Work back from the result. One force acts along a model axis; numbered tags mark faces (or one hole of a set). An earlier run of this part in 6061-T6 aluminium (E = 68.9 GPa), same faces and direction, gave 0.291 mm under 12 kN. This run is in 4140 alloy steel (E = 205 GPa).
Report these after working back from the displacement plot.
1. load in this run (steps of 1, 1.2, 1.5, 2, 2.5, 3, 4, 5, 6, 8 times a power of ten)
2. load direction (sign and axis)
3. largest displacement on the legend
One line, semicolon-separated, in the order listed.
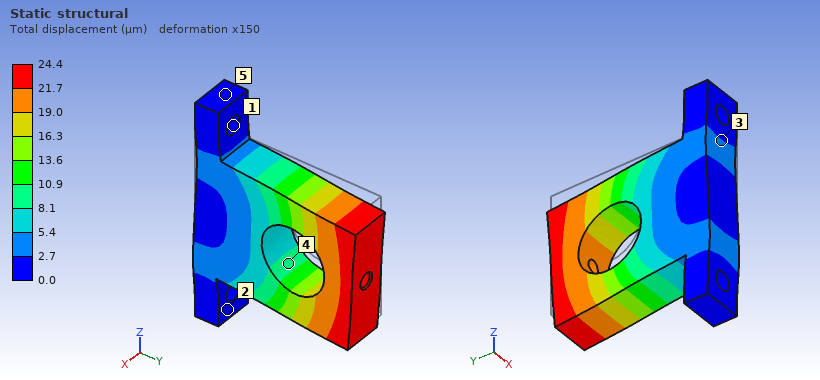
3 kN; -Z; 24.4 µm
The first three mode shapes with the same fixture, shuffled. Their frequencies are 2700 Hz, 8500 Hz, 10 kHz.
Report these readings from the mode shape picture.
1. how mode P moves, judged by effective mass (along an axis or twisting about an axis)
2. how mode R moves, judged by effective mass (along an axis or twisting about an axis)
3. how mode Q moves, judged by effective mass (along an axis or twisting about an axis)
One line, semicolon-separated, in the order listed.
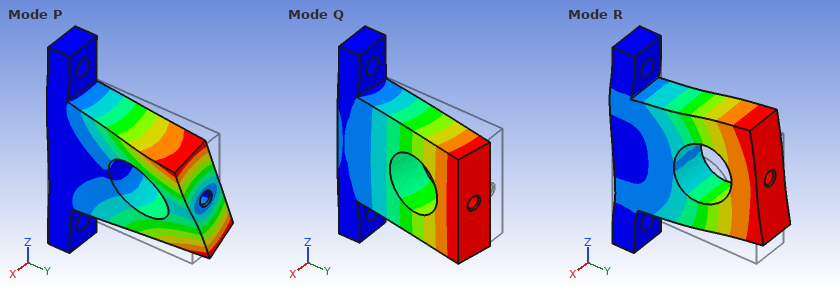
twisting about Y; along Z; along X
